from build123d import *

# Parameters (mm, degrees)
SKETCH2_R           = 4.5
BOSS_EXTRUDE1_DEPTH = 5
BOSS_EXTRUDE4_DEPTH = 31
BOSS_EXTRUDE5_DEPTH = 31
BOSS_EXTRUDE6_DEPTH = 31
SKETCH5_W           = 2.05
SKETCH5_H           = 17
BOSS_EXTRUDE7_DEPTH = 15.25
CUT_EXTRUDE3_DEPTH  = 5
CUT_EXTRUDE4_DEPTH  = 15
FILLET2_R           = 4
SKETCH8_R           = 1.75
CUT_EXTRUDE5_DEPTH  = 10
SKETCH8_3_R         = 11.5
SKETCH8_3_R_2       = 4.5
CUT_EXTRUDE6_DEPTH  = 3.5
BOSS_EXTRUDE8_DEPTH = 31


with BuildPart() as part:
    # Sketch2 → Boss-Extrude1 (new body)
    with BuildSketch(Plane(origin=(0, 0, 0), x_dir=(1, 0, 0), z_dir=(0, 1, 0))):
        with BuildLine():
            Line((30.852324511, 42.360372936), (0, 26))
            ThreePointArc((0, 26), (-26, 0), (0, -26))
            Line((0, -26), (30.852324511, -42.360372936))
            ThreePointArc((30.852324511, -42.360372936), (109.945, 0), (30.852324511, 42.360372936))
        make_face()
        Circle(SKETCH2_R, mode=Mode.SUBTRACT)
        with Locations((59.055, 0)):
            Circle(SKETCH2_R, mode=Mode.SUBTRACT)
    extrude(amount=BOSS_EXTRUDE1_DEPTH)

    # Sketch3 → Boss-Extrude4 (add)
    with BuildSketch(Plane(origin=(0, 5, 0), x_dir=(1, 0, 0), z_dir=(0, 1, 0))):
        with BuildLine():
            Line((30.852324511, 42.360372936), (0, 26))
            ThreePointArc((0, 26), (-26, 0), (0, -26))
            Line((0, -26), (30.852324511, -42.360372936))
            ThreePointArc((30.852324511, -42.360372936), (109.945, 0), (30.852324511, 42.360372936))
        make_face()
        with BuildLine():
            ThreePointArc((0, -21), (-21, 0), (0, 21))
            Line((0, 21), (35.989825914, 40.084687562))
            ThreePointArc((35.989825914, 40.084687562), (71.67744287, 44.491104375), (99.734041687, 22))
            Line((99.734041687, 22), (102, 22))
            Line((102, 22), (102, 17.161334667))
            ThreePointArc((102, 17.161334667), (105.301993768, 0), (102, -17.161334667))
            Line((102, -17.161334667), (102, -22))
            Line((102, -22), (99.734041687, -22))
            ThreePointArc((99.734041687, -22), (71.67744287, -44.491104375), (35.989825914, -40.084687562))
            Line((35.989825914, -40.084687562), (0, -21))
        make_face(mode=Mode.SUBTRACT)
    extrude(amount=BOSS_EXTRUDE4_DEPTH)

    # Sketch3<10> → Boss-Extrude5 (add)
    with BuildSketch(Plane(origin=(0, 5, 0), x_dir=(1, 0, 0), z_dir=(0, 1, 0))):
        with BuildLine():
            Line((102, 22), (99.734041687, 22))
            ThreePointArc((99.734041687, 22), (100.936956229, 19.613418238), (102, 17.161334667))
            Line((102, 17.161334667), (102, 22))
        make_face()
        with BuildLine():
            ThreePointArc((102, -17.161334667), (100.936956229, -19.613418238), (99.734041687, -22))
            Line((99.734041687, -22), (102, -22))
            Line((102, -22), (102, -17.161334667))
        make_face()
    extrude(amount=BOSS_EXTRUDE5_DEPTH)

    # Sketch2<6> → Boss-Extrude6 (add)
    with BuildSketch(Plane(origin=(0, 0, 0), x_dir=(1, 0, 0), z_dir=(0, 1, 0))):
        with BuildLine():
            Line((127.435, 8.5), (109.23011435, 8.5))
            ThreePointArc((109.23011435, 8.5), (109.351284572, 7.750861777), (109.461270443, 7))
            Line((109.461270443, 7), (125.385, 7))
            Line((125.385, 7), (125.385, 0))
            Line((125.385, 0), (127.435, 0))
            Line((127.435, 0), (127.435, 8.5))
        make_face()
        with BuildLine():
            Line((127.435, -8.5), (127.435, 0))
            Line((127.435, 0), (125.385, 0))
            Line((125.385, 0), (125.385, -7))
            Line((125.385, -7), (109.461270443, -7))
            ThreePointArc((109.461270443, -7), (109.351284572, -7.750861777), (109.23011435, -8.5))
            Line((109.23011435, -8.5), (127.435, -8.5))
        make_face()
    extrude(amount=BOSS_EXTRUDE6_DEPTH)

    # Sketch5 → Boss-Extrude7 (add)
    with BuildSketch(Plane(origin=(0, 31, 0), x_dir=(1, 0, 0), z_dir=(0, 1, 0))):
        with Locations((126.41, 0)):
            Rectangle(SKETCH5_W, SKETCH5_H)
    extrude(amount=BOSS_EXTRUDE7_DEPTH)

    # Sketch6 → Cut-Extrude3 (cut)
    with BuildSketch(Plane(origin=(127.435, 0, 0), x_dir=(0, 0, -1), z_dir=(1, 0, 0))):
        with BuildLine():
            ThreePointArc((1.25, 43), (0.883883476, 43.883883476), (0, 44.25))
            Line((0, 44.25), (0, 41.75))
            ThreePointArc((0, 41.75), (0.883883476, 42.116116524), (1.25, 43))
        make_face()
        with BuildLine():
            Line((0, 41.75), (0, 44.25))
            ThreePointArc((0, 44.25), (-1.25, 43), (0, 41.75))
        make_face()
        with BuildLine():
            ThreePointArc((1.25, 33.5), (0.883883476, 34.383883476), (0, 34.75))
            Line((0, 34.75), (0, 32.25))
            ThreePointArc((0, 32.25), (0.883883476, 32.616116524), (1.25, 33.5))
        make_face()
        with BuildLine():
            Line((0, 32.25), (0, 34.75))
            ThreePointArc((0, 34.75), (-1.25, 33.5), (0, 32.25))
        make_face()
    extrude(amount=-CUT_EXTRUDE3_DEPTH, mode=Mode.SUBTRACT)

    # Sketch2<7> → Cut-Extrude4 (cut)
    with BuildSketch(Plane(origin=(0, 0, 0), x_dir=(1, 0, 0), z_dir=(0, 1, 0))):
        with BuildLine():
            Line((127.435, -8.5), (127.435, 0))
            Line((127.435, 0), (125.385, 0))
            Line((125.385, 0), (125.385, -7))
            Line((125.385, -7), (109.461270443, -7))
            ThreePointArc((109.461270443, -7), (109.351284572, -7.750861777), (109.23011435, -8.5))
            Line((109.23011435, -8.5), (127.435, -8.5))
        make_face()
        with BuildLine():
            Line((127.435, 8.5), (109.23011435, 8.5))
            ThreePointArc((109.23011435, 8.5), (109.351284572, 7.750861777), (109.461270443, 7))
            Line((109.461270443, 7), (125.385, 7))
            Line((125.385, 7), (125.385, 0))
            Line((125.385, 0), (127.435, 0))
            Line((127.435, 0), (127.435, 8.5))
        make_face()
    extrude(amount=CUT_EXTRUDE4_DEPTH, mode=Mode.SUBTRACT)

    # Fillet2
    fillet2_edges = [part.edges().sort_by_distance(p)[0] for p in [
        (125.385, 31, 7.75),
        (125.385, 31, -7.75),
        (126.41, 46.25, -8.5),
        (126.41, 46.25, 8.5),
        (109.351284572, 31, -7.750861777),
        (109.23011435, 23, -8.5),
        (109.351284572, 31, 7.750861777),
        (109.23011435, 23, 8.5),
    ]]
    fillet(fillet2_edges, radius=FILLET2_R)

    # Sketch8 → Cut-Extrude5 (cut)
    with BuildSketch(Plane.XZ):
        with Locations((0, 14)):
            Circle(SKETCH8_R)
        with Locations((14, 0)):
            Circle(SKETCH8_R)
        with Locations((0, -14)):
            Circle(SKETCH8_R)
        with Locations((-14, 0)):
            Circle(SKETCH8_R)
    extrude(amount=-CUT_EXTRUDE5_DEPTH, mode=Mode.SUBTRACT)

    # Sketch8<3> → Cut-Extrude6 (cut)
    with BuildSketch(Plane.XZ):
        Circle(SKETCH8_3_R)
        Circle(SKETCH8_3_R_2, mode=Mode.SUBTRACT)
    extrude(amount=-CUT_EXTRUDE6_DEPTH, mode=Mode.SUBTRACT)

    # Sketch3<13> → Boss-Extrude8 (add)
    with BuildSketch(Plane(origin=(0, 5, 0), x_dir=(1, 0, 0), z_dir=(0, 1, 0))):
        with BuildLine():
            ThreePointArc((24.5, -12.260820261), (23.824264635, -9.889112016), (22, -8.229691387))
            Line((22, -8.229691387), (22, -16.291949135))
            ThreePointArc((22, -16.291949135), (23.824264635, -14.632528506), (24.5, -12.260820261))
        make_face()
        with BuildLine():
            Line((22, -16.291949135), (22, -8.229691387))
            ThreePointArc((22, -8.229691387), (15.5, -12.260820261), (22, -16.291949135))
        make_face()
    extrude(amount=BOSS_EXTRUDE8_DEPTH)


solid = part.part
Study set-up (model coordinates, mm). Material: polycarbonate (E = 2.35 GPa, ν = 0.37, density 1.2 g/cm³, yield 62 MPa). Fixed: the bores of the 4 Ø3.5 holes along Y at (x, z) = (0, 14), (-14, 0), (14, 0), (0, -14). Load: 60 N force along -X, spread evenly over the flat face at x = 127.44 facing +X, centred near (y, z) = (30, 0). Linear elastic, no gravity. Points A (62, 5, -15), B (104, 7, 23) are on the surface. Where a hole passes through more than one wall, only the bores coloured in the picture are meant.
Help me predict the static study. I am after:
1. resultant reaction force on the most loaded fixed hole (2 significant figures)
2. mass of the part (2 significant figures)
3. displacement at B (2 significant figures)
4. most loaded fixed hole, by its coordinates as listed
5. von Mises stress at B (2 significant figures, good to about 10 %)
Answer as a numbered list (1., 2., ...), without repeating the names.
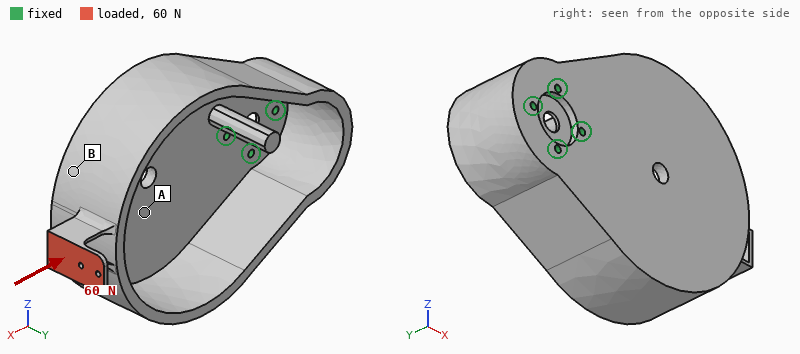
1. 43 N
2. 120 g
3. 0.55 mm
4. (-14, 0)
5. 2.1 MPa
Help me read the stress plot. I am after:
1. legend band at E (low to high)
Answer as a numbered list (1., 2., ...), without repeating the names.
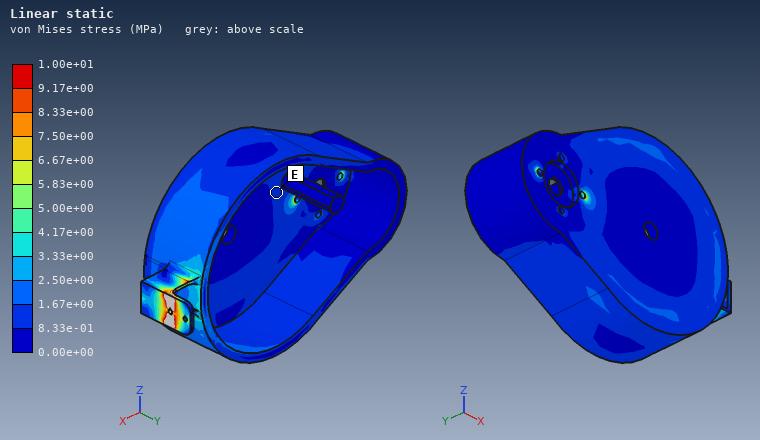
1. 8.33e-01 to 1.67e+00 MPa
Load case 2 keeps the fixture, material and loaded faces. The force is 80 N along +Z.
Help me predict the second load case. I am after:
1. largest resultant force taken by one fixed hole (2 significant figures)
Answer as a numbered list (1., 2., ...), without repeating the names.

1. 220 N
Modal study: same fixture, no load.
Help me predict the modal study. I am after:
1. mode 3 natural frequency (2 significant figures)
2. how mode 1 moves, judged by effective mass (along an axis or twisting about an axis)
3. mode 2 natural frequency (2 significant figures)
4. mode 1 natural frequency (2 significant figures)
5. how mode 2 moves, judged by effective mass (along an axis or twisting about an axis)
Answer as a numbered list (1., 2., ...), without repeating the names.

1. 490 Hz
2. along Y
3. 340 Hz
4. 170 Hz
5. along Z
